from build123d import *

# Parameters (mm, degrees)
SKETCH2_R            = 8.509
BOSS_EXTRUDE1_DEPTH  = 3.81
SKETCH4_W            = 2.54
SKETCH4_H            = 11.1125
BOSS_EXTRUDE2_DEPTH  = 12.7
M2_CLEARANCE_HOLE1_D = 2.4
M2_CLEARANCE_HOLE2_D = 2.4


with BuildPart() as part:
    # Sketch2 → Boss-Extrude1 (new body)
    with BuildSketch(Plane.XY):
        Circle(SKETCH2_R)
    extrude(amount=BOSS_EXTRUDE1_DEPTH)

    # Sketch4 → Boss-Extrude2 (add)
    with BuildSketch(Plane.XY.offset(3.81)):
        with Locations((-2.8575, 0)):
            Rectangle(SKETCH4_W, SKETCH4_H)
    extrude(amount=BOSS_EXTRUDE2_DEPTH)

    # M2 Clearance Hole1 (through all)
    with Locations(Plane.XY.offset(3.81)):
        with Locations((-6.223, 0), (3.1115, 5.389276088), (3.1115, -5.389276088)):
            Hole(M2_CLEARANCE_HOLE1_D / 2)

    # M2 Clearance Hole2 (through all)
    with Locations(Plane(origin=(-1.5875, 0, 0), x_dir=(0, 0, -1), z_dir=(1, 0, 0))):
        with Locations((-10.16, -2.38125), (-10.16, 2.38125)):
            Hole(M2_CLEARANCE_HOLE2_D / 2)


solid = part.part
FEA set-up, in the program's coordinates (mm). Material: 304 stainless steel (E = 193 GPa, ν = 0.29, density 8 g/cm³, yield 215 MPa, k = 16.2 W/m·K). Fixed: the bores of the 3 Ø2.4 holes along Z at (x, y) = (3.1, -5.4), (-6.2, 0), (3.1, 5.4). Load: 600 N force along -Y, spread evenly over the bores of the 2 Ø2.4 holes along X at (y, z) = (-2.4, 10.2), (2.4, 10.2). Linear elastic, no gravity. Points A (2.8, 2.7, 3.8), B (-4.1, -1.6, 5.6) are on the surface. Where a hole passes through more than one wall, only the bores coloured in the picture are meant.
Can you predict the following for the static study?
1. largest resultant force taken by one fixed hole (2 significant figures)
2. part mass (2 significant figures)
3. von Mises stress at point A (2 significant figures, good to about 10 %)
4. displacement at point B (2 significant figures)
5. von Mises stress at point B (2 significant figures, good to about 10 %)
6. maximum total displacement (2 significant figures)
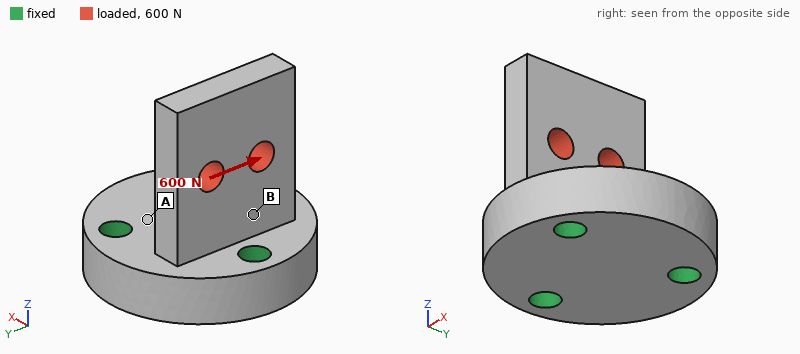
330 N
9.2 g
20 MPa
2.3 µm
45 MPa
11 µm
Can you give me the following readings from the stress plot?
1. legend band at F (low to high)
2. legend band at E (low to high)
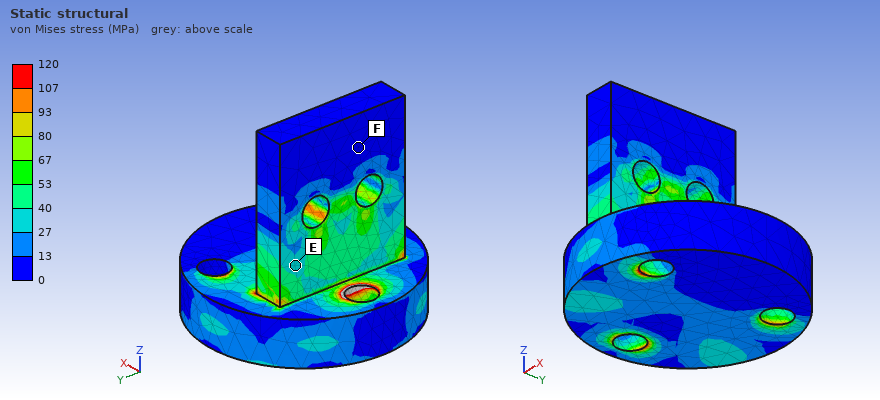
0 to 13 MPa
27 to 40 MPa
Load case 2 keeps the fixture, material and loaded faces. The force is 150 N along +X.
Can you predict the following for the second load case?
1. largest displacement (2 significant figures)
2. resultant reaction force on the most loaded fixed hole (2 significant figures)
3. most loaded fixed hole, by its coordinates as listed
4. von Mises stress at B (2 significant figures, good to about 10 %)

16 µm
170 N
(-6.2, 0)
53 MPa
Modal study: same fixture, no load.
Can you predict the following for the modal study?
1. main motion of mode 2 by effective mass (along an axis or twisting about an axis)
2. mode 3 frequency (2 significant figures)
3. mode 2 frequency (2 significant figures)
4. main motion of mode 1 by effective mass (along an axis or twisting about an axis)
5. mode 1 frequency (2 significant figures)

along Y
26 kHz
25 kHz
along X
11 kHz
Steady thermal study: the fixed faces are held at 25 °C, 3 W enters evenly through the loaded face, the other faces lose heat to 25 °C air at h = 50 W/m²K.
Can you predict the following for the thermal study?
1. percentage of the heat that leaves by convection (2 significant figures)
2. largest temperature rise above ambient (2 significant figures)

24 %
50 K
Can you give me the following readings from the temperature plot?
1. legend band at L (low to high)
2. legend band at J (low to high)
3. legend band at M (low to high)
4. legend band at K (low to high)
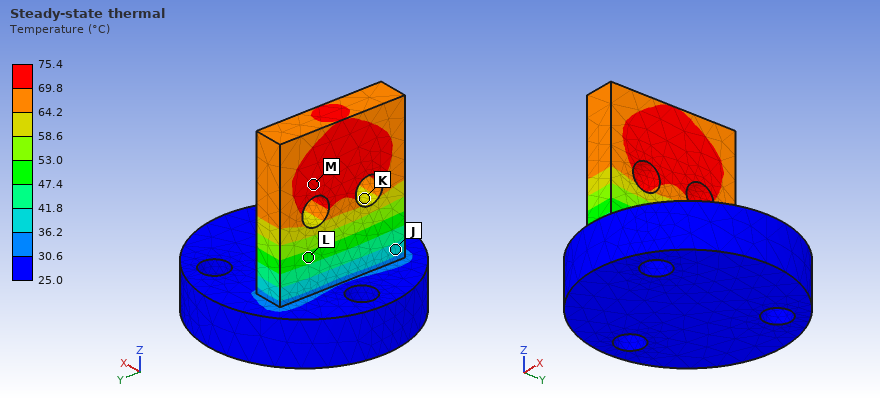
47.4 to 53.0 °C
36.2 to 41.8 °C
69.8 to 75.4 °C
58.6 to 64.2 °C
